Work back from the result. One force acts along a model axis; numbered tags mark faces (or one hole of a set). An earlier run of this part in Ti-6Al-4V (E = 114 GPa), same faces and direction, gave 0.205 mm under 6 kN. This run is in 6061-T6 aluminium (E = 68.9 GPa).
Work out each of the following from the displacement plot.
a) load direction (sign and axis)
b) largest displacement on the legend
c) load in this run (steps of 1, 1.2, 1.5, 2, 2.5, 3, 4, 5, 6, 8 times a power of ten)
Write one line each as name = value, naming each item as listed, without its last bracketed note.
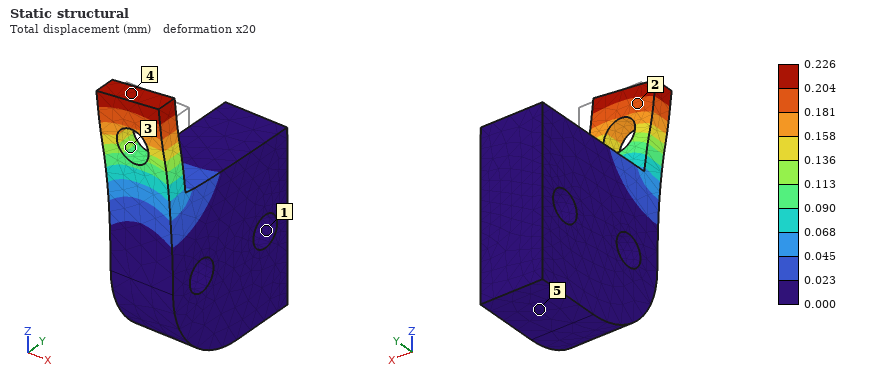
load direction = -X
largest displacement on the legend = 0.226 mm
load in this run = 4 kN
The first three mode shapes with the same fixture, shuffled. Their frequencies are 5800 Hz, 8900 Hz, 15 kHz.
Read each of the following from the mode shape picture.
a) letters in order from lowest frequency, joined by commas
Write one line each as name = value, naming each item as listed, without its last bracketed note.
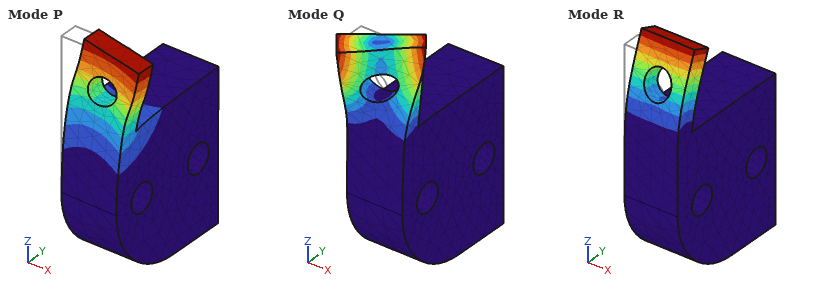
letters in order from lowest frequency, joined by commas = R, P, Q
